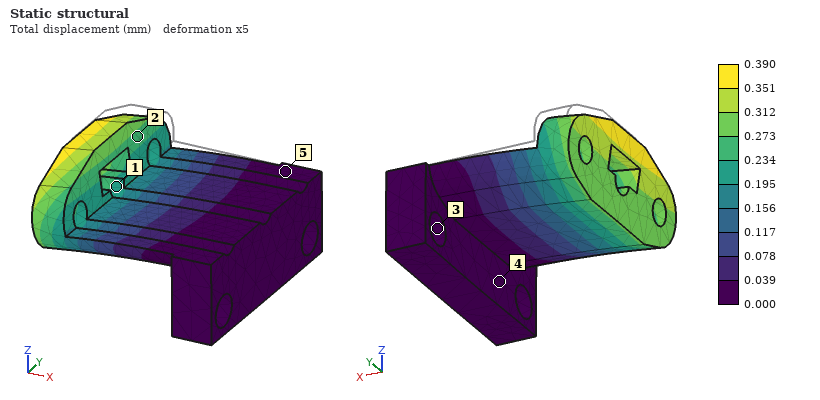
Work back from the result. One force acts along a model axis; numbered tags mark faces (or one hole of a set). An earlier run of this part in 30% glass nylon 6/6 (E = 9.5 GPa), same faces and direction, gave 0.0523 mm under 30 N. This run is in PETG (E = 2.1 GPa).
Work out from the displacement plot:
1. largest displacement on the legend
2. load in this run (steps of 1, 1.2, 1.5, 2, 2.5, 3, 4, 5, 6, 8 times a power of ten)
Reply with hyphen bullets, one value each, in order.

- 0.390 mm
- 50 N
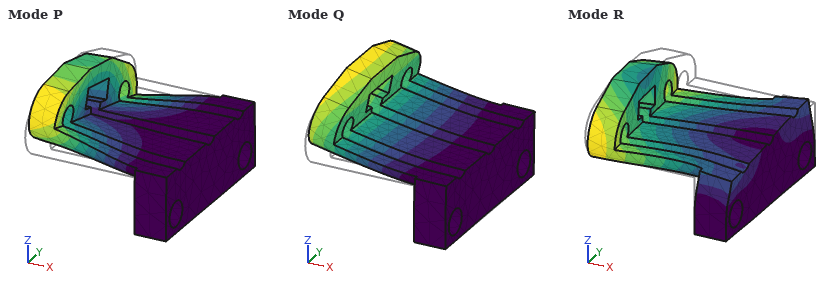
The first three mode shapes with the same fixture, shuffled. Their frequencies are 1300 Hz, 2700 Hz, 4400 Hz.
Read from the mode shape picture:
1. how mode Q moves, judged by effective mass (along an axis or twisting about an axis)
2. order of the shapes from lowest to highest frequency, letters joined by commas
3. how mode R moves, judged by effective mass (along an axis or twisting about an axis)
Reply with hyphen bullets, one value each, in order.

- along Z
- Q, P, R
- along Y
